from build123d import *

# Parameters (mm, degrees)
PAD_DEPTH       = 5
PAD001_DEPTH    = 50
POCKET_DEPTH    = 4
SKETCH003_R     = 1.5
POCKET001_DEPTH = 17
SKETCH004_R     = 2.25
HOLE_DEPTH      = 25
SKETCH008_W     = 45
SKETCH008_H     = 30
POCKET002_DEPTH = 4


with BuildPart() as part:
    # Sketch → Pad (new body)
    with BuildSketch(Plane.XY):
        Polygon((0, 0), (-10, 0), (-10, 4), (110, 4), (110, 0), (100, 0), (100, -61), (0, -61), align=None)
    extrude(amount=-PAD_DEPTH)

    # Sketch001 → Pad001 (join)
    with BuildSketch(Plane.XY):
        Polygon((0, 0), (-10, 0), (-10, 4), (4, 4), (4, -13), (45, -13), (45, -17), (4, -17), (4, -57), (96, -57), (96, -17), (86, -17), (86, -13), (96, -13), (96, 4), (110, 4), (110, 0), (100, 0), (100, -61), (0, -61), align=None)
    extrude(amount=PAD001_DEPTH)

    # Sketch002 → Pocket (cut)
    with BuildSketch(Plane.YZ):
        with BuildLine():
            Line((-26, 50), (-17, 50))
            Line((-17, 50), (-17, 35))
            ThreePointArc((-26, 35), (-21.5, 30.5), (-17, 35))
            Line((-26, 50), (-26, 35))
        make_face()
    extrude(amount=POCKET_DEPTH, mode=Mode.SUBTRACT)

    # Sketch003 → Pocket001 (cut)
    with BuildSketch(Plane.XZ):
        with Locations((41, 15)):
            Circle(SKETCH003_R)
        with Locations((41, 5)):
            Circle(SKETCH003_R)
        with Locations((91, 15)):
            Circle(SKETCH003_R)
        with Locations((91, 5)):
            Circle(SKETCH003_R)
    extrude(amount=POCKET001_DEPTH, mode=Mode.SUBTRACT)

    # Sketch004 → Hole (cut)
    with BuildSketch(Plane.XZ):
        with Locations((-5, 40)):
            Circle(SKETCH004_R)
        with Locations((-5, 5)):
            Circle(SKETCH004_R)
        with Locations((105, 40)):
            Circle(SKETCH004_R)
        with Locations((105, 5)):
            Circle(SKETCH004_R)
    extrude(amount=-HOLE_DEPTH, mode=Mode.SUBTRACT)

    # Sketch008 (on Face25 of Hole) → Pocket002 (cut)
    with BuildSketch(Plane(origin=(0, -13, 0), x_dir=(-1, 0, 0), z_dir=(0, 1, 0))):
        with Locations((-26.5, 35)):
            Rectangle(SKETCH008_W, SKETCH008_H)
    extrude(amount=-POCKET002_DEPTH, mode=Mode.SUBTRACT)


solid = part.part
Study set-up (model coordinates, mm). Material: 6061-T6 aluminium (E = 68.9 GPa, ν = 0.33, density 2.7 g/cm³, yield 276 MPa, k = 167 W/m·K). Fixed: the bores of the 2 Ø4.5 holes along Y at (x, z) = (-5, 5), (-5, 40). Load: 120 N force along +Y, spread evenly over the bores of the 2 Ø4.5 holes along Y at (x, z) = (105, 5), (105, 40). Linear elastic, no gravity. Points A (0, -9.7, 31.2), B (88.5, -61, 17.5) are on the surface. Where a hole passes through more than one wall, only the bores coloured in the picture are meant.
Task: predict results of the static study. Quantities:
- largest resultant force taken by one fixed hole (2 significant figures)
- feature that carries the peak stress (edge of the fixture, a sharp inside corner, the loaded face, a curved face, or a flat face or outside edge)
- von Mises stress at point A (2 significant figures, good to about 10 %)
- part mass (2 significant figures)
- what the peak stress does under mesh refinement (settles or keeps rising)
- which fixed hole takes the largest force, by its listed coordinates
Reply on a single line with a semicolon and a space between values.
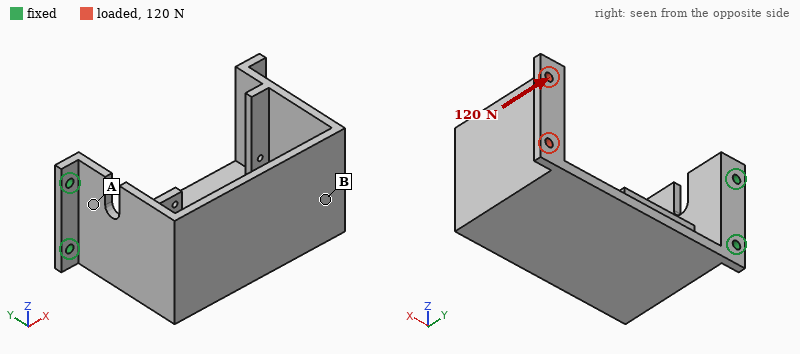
91 N; edge of the fixture; 43 MPa; 230 g; keeps rising; (-5, 5)
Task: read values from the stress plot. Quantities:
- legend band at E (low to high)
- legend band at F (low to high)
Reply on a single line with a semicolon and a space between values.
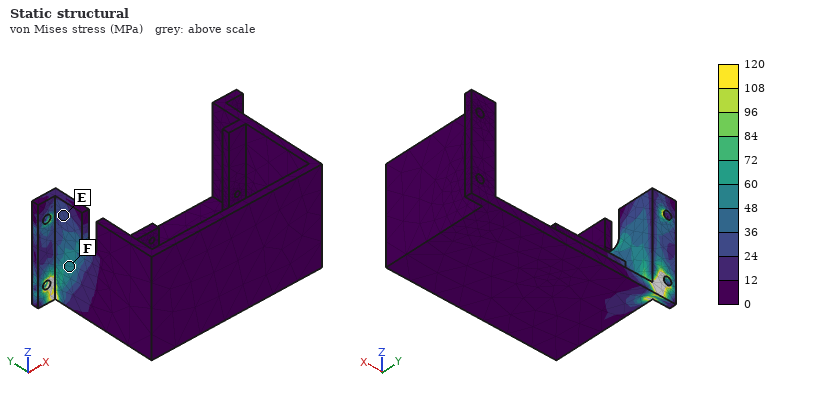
24 to 36 MPa; 48 to 60 MPa
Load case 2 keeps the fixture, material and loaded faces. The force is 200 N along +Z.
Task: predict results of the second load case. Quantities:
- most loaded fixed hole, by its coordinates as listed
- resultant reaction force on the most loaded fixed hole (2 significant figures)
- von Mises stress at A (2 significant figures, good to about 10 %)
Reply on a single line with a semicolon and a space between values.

(-5, 40); 680 N; 27 MPa
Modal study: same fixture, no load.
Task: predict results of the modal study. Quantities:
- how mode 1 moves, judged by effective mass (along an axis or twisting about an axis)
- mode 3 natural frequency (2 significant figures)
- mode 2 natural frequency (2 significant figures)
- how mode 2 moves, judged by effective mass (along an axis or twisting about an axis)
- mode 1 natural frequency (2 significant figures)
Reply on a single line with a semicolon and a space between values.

along Y; 720 Hz; 290 Hz; along Z; 150 Hz
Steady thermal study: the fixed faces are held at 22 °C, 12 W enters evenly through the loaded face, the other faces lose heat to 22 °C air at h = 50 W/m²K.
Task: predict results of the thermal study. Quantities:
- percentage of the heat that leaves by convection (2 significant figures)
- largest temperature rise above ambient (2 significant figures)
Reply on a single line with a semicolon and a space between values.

82 %; 18 K
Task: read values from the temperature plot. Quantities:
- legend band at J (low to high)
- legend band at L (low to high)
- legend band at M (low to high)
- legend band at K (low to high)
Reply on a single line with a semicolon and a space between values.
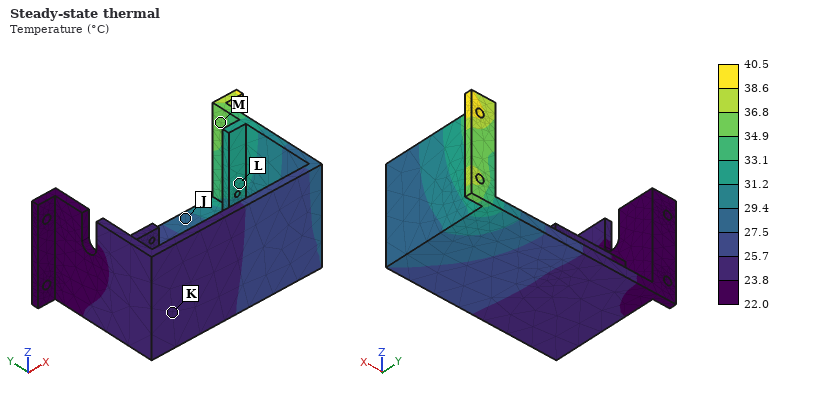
27.5 to 29.4 °C; 31.2 to 33.1 °C; 34.9 to 36.8 °C; 23.8 to 25.7 °C
